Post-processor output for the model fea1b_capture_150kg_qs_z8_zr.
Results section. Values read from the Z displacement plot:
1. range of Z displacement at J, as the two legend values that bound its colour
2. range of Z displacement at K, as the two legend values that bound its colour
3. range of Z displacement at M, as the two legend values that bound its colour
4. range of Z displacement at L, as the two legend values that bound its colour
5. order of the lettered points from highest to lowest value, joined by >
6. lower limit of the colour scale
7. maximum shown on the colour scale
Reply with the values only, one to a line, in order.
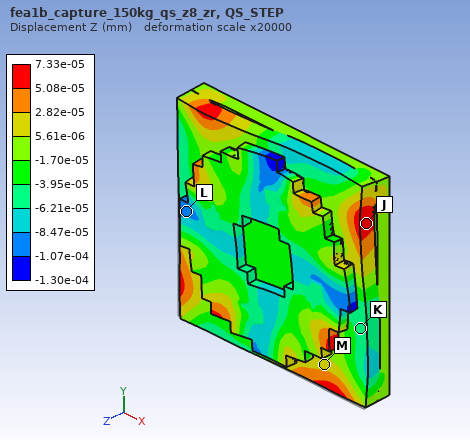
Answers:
5.08e-05 to 7.33e-05 mm
-6.21e-05 to -3.95e-05 mm
5.61e-06 to 2.82e-05 mm
-1.07e-04 to -8.47e-05 mm
J > M > K > L
-1.30e-04 mm
7.33e-05 mm
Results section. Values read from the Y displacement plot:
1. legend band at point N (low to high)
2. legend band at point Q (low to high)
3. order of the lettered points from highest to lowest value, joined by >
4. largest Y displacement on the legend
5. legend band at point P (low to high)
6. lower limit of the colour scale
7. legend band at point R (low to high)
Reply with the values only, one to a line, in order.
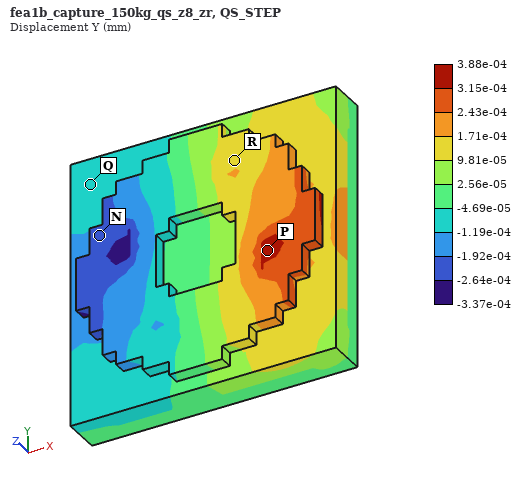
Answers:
-2.64e-04 to -1.92e-04 mm
-1.19e-04 to -4.69e-05 mm
P > R > Q > N
3.88e-04 mm
3.15e-04 to 3.88e-04 mm
-3.37e-04 mm
9.81e-05 to 1.71e-04 mm
